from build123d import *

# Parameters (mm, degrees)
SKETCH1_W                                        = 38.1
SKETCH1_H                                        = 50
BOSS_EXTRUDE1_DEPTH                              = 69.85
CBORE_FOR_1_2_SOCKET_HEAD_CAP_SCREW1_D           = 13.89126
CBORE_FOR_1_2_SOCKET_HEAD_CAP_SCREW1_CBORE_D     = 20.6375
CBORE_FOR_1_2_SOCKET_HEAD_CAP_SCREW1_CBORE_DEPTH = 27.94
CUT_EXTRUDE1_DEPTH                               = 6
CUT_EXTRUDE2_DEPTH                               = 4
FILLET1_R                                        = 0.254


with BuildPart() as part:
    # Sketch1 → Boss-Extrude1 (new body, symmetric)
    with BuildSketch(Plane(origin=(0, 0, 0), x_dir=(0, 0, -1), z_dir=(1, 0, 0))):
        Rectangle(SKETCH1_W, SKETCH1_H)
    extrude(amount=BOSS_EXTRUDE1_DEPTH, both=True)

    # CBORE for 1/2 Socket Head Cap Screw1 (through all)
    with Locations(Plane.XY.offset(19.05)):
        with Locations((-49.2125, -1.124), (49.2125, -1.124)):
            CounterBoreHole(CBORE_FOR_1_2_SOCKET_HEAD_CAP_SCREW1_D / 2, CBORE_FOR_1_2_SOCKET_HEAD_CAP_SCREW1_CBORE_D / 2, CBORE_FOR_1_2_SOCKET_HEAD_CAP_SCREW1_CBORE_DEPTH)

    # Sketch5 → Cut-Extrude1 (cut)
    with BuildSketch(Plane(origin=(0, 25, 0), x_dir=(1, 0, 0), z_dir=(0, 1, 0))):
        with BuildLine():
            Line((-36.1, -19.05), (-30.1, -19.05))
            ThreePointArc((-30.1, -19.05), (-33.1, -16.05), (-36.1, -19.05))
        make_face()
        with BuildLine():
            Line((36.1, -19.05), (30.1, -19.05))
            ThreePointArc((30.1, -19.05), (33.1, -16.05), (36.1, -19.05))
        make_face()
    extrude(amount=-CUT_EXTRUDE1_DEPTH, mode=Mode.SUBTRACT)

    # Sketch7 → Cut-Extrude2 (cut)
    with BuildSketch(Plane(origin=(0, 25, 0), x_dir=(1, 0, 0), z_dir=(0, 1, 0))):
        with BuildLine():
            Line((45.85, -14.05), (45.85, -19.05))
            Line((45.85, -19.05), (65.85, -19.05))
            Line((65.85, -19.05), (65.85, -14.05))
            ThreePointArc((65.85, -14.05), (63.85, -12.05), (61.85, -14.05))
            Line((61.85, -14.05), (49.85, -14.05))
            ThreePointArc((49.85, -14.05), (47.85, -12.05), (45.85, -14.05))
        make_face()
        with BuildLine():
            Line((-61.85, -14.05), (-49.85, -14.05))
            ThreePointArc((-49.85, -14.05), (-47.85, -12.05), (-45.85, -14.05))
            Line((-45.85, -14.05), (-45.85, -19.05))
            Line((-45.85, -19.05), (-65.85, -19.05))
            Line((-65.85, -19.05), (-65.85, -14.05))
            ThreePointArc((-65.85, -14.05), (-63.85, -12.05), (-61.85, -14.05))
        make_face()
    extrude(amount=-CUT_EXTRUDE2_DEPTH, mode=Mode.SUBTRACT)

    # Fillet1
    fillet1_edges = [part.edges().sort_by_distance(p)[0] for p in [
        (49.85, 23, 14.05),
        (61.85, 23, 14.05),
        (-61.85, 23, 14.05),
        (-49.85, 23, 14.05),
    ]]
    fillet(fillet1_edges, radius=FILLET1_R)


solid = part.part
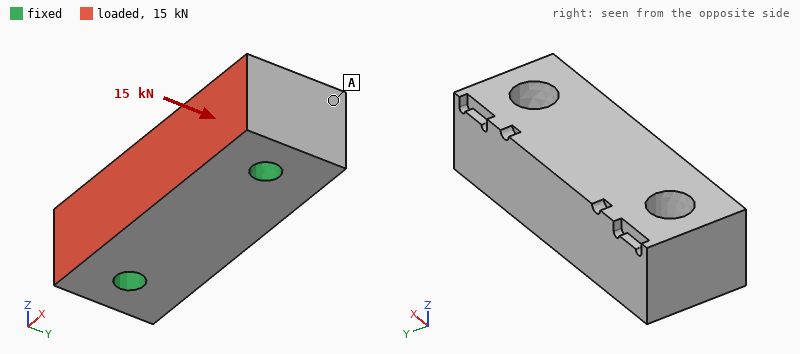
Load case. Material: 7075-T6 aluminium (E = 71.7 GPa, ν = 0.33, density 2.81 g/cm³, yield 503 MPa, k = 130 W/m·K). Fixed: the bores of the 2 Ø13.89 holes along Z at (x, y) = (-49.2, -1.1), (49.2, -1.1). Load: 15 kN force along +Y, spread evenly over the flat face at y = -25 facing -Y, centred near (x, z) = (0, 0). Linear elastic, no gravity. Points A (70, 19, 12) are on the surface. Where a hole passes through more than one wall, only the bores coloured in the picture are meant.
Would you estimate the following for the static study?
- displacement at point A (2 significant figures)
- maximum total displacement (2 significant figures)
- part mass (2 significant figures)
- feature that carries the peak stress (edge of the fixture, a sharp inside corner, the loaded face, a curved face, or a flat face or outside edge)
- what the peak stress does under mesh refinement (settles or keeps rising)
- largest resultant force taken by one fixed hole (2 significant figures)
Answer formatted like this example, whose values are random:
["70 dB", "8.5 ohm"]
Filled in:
["32 µm", "47 µm", "680 g", "edge of the fixture", "keeps rising", "7.5 kN"]
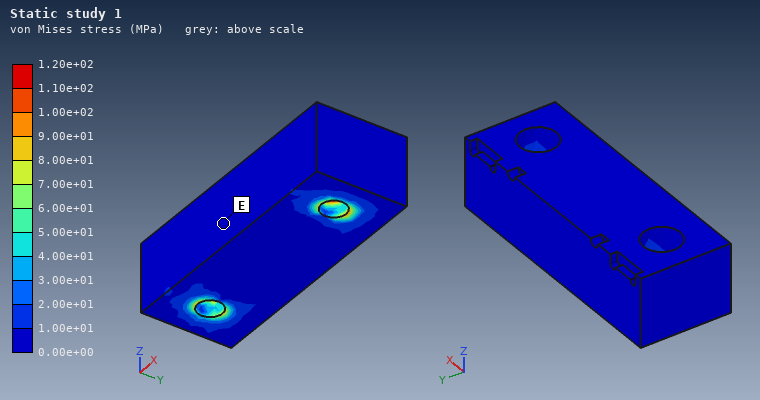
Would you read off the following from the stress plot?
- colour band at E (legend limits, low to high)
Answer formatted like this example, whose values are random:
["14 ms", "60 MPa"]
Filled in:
["0.00e+00 to 1.00e+01 MPa"]
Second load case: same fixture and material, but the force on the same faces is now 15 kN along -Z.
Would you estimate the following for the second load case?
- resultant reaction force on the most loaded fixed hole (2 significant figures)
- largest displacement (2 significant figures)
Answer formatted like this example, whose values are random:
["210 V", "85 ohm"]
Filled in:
["7.9 kN", "76 µm"]
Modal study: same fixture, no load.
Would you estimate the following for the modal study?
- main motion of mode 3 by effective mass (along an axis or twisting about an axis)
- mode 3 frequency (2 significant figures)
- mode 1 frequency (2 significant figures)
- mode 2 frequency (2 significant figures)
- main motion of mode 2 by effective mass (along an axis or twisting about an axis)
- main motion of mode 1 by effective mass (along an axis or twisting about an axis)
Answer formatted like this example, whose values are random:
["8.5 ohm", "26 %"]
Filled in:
["twisting about Z", "8800 Hz", "3800 Hz", "8000 Hz", "along Z", "along Y"]
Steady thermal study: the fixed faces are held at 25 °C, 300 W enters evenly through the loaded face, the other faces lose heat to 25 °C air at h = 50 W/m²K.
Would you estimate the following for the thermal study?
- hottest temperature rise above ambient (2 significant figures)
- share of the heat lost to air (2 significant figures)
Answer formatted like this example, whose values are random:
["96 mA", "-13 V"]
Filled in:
["31 K", "7.5 %"]
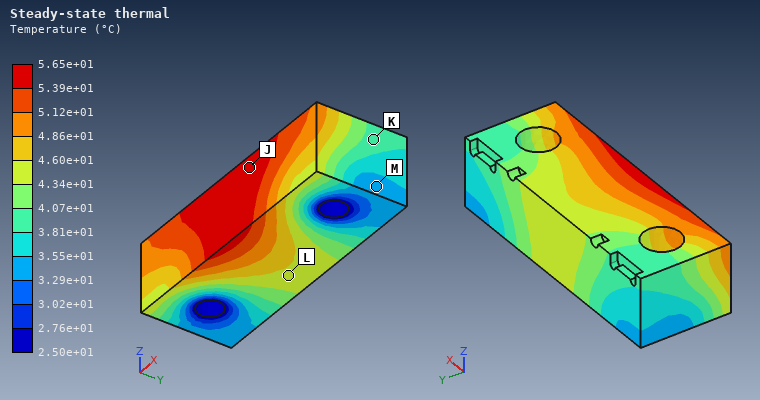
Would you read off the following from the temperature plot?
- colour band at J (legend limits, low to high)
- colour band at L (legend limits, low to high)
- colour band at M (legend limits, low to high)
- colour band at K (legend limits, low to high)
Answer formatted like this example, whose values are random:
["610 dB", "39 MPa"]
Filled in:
["5.39e+01 to 5.65e+01 °C", "4.34e+01 to 4.60e+01 °C", "3.29e+01 to 3.55e+01 °C", "3.81e+01 to 4.07e+01 °C"]
